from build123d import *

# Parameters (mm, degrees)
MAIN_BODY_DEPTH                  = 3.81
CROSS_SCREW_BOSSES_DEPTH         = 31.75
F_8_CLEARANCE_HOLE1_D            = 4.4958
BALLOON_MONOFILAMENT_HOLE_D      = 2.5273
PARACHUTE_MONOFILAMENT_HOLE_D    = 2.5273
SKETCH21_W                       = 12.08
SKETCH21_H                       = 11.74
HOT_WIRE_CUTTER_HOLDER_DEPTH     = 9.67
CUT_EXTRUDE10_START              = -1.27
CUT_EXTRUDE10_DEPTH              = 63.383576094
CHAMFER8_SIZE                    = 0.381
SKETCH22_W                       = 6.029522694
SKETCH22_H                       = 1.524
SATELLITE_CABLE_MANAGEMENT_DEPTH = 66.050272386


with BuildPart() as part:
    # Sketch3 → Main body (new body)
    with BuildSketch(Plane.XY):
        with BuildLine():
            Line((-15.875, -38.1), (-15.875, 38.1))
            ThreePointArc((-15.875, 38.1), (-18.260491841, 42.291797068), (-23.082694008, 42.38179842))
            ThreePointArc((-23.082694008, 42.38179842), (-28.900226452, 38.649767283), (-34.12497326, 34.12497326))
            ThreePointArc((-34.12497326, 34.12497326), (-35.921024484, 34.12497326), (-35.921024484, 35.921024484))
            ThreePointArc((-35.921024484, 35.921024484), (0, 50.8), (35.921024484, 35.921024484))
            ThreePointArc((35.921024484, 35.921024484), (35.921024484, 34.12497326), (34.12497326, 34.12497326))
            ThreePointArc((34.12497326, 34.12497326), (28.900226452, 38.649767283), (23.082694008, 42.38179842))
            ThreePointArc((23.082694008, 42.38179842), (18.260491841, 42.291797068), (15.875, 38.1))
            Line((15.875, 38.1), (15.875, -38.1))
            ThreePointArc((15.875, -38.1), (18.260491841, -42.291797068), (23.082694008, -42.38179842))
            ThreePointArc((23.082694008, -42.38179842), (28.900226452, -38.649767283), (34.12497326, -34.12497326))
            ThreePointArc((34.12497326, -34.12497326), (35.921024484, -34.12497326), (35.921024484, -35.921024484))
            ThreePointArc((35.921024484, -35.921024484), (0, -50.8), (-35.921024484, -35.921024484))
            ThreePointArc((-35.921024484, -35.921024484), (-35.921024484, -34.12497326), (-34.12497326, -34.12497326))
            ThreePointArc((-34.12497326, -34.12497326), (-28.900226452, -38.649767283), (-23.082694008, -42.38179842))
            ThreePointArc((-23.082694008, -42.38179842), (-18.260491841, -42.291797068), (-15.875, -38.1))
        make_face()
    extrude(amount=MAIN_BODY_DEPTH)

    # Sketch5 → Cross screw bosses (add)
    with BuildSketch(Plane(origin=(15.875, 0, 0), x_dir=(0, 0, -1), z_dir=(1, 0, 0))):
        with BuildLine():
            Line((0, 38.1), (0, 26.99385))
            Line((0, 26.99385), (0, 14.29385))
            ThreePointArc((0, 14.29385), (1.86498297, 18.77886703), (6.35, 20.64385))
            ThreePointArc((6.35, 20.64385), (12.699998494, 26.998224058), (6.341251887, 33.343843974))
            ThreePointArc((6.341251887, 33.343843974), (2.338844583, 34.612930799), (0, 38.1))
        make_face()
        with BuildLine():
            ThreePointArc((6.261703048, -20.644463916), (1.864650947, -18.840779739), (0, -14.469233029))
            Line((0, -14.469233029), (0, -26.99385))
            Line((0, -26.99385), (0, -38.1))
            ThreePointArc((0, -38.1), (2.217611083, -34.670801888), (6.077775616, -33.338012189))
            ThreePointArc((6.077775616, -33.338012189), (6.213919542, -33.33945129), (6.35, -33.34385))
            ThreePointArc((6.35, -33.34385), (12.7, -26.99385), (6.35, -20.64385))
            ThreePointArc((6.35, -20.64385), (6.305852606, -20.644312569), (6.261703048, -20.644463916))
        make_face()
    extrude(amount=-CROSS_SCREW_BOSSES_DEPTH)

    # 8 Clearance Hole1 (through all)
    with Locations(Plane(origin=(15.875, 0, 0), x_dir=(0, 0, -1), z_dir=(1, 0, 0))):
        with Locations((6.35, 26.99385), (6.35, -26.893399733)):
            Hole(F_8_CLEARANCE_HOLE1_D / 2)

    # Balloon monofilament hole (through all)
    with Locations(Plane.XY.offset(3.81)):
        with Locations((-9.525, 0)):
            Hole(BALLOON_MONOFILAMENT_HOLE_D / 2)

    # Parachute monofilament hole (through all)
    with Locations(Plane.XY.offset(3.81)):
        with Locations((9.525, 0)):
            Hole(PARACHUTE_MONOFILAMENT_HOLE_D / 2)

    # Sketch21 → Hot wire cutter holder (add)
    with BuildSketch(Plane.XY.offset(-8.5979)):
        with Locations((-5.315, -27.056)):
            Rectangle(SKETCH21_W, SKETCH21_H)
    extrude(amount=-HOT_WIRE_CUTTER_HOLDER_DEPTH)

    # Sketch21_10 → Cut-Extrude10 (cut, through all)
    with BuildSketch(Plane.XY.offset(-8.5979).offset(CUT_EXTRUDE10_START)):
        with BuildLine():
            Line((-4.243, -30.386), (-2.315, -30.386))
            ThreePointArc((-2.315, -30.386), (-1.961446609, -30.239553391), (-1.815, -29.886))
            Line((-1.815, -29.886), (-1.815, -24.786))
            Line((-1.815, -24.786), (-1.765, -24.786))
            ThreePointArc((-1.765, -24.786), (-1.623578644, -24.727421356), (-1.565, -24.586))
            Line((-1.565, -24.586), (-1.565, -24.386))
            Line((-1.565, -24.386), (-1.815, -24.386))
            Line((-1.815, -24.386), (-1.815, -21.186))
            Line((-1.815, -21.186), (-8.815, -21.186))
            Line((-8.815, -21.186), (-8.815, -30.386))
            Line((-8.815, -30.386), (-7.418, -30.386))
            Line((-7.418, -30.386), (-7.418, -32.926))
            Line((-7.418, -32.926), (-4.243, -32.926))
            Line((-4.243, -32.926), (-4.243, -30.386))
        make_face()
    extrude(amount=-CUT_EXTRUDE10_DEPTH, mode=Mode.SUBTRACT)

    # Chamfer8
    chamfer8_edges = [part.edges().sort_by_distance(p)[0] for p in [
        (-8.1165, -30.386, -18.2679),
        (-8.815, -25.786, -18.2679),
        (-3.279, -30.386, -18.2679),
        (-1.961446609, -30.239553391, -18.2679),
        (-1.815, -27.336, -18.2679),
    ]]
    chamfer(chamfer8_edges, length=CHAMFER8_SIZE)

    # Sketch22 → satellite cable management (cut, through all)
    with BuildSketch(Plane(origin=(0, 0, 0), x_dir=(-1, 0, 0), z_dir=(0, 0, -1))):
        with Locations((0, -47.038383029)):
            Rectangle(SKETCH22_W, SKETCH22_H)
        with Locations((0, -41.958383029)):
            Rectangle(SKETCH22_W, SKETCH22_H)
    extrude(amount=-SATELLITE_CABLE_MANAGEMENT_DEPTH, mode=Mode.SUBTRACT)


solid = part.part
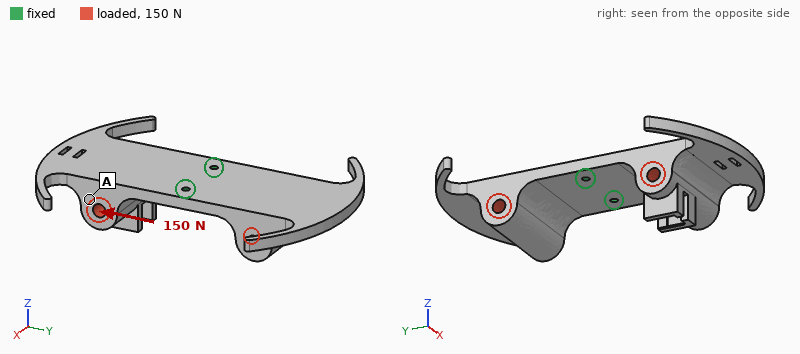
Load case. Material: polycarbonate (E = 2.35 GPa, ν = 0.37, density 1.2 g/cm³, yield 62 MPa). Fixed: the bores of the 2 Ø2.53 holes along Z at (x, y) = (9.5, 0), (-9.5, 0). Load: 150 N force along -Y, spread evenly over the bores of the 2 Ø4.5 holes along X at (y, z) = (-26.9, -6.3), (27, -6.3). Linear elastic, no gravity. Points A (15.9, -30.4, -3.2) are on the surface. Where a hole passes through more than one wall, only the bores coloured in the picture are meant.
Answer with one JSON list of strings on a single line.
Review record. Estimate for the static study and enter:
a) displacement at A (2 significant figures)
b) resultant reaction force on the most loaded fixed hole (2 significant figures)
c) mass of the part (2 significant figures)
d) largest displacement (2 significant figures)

["0.81 mm", "75 N", "27 g", "1.5 mm"]
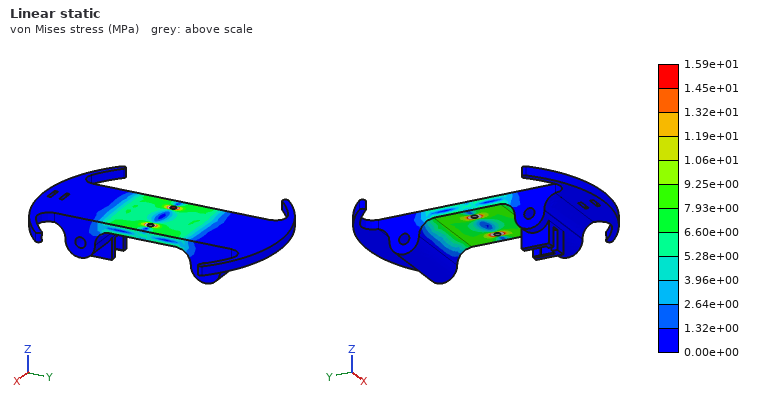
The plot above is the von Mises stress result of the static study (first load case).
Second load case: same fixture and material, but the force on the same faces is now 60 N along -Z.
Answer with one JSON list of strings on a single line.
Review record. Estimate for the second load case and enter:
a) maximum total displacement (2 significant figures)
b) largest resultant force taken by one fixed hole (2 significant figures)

["1.1 mm", "30 N"]
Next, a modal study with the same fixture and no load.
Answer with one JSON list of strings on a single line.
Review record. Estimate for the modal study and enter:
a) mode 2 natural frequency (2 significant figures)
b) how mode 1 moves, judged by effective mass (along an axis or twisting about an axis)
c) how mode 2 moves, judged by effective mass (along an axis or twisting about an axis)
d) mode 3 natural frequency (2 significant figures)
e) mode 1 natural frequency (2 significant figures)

["280 Hz", "twisting about X", "along Z", "830 Hz", "250 Hz"]
